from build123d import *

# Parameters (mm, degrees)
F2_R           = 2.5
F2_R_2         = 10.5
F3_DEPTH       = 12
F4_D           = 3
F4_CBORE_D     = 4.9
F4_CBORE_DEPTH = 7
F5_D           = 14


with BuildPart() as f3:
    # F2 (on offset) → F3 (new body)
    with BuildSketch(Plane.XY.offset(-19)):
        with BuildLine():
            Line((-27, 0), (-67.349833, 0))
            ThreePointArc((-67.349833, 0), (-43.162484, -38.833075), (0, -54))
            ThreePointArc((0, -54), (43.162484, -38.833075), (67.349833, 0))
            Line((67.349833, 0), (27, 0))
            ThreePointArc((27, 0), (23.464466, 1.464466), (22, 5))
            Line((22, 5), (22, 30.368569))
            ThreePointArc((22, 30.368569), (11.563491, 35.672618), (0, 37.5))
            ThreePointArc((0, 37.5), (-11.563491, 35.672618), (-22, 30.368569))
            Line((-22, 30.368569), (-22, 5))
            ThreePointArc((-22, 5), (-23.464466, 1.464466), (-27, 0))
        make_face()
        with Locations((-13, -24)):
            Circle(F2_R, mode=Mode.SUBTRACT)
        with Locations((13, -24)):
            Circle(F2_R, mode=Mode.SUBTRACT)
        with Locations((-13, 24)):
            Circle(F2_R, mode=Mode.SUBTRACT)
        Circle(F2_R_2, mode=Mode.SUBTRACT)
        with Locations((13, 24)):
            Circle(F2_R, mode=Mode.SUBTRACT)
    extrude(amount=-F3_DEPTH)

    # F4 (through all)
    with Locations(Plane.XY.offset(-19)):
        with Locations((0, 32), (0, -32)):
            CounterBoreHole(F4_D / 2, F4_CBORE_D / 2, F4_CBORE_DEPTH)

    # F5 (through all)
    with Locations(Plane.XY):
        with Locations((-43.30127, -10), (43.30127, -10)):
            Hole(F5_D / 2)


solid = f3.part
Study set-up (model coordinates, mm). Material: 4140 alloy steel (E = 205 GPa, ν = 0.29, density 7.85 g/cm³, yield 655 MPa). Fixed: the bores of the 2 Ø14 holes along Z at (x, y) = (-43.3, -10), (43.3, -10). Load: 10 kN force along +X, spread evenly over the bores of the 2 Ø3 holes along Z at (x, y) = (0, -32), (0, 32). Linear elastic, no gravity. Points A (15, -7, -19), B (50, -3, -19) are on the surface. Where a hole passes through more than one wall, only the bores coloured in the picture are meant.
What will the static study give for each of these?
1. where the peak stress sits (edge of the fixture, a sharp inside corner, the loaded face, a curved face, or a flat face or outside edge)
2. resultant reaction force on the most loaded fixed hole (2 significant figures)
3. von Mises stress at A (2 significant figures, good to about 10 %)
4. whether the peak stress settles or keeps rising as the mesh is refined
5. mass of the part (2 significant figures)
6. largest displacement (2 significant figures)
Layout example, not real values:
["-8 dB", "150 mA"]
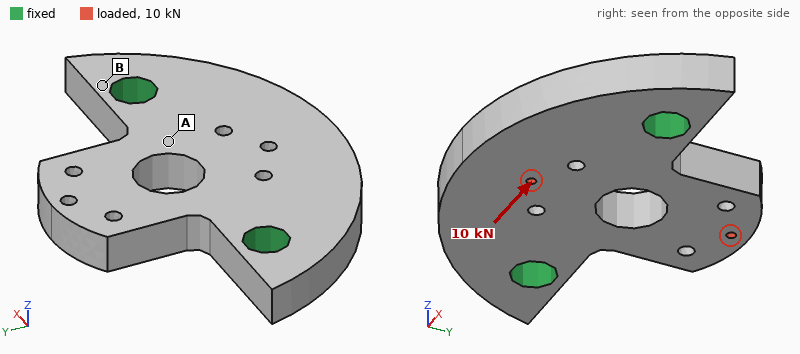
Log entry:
["a sharp inside corner", "5.3 kN", "19 MPa", "keeps rising", "590 g", "20 µm"]
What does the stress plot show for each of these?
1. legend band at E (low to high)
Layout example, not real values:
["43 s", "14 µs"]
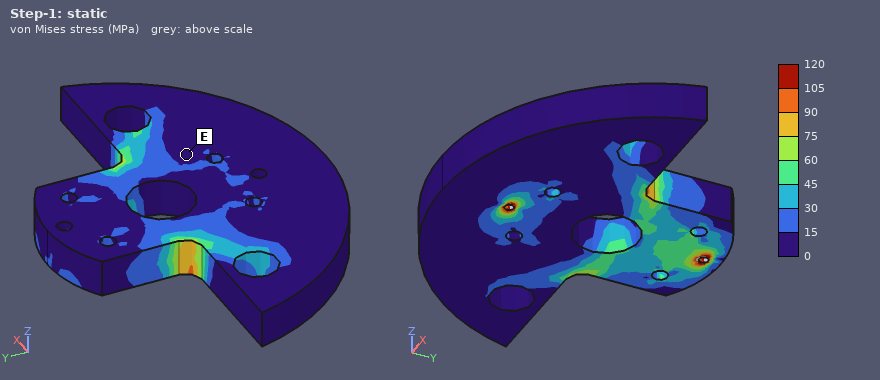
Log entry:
["0 to 15 MPa"]
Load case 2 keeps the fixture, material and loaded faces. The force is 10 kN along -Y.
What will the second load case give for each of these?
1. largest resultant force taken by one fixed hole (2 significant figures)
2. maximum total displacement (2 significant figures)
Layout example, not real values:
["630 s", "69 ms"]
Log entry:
["5.2 kN", "37 µm"]
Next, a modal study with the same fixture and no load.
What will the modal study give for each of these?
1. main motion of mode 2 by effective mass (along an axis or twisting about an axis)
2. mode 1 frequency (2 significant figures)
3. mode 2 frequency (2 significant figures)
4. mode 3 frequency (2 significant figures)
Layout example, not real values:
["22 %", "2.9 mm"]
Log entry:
["along Z", "3000 Hz", "5000 Hz", "9200 Hz"]
